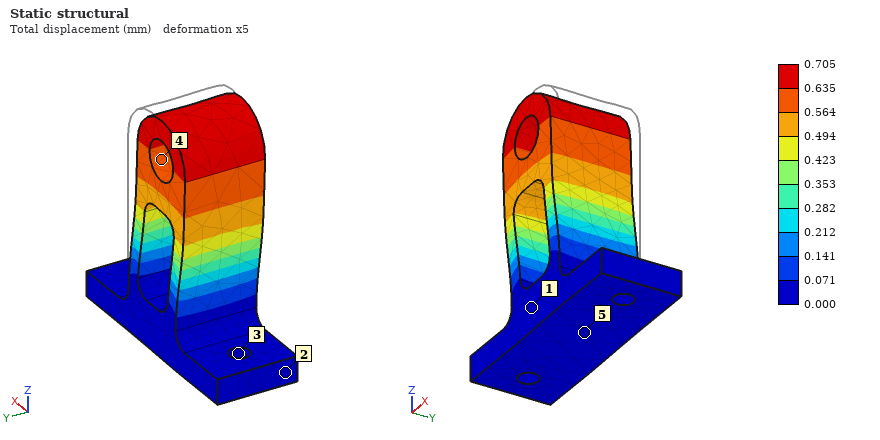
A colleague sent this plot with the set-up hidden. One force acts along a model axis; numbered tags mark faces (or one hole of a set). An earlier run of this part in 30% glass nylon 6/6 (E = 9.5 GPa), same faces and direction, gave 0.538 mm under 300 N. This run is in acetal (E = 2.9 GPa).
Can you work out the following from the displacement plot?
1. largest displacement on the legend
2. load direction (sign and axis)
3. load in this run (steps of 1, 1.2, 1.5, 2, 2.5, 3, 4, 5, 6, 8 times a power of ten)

0.705 mm
-X
120 N
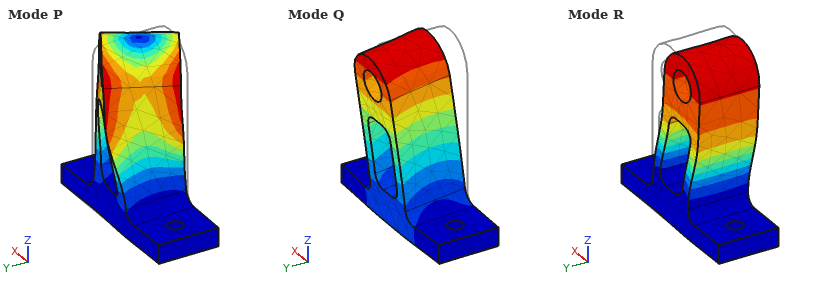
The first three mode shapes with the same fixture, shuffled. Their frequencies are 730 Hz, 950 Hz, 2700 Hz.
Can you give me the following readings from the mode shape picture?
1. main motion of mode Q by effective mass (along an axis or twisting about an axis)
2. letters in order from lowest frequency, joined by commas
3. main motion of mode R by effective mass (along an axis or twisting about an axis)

along Y
Q, R, P
along X
